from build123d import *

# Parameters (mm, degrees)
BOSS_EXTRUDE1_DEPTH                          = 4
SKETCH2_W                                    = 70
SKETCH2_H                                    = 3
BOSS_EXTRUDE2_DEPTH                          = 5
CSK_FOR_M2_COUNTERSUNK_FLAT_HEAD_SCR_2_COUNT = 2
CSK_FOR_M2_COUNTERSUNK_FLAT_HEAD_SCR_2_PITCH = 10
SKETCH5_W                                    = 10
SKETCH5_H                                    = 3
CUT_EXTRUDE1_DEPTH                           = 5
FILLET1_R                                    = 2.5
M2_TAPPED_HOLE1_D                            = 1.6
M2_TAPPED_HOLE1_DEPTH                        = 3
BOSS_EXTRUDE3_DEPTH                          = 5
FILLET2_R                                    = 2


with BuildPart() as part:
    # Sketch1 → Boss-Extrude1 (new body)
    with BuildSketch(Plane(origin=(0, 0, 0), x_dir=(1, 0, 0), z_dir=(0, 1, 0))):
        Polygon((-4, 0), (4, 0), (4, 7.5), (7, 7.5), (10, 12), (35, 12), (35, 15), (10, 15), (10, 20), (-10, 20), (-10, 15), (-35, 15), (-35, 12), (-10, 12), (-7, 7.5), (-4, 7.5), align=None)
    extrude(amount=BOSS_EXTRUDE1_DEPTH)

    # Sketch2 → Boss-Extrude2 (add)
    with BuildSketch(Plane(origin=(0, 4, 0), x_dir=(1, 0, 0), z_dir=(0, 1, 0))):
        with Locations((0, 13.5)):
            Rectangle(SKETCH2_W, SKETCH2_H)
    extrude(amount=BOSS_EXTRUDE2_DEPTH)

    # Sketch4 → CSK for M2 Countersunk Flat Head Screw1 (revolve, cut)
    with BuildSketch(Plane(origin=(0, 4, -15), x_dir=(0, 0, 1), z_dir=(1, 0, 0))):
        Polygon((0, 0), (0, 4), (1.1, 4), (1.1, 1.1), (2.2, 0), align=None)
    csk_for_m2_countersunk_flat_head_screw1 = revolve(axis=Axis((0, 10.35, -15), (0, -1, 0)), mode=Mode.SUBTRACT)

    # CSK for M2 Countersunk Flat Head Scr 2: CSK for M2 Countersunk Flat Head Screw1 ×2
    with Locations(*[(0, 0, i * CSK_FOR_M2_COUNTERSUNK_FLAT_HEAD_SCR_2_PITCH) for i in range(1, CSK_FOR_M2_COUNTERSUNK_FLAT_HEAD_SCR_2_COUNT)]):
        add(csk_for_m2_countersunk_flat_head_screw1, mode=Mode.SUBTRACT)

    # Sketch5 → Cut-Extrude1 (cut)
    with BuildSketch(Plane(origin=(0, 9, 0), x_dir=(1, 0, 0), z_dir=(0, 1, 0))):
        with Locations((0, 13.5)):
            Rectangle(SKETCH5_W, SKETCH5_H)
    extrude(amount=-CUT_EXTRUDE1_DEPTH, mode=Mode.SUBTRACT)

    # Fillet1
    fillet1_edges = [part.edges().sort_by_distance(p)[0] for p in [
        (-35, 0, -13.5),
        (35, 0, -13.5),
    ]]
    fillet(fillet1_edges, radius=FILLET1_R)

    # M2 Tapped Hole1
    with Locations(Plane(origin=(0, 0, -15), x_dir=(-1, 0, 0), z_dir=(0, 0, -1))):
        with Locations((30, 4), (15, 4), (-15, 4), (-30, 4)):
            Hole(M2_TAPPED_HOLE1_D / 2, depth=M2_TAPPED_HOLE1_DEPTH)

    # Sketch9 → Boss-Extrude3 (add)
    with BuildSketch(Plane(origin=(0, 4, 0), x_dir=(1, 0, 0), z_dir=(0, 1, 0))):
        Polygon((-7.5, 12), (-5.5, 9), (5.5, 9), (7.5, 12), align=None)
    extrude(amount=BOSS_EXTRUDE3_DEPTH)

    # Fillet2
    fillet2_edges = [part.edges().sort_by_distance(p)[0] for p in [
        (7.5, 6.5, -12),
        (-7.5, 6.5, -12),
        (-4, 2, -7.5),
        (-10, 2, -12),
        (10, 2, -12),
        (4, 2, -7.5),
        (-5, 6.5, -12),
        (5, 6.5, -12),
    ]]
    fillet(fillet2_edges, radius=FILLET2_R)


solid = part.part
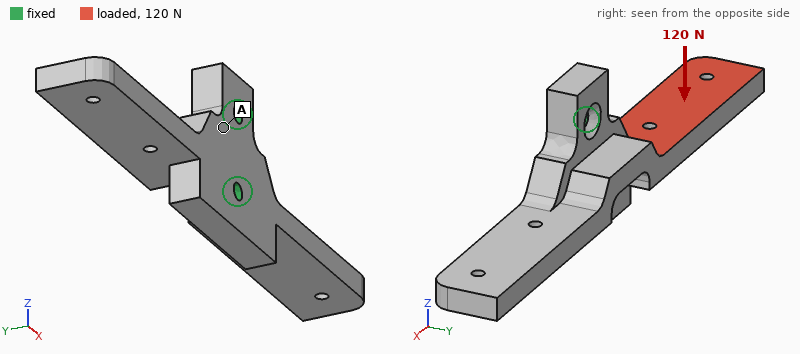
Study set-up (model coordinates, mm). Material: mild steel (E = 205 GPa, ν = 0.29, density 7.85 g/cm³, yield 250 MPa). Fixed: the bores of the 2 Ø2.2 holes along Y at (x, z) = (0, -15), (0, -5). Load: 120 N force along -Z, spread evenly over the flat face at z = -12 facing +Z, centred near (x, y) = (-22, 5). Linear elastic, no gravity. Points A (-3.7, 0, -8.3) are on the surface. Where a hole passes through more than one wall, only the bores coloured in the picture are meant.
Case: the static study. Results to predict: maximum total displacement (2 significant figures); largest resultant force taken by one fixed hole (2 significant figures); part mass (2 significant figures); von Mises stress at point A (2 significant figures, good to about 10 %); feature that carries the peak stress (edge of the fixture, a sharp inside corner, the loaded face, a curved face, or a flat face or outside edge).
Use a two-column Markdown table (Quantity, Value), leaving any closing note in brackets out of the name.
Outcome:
| Quantity | Value |
|---|---|
| maximum total displacement | 82 µm |
| largest resultant force taken by one fixed hole | 260 N |
| part mass | 22 g |
| von Mises stress at point A | 17 MPa |
| feature that carries the peak stress | the loaded face |
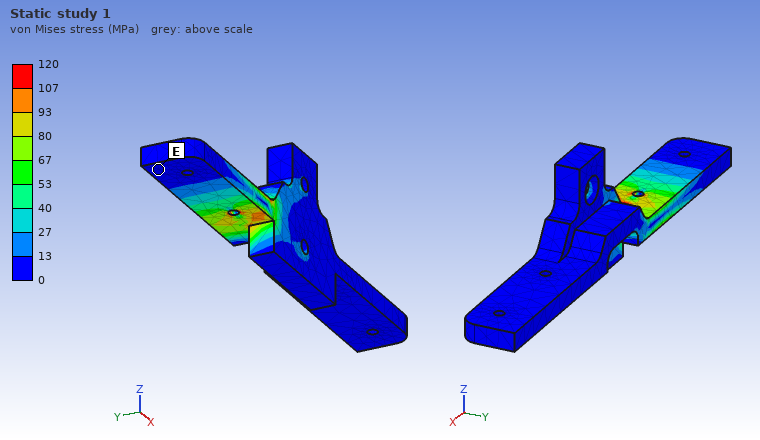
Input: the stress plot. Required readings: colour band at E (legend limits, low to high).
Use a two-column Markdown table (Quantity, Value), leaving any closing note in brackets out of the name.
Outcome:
| Quantity | Value |
|---|---|
| colour band at E | 0 to 13 MPa |
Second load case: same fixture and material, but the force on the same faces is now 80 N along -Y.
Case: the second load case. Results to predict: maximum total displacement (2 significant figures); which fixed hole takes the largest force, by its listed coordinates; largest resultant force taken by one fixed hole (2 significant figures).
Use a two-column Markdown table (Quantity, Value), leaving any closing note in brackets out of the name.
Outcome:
| Quantity | Value |
|---|---|
| maximum total displacement | 27 µm |
| which fixed hole takes the largest force, by its listed coordinates | (0, -15) |
| largest resultant force taken by one fixed hole | 70 N |
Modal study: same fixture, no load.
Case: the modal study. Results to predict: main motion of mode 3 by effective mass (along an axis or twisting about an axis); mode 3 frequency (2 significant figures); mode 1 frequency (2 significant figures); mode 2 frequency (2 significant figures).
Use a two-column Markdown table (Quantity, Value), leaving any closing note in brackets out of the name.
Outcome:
| Quantity | Value |
|---|---|
| main motion of mode 3 by effective mass | twisting about Z |
| mode 3 frequency | 3900 Hz |
| mode 1 frequency | 3300 Hz |
| mode 2 frequency | 3400 Hz |
